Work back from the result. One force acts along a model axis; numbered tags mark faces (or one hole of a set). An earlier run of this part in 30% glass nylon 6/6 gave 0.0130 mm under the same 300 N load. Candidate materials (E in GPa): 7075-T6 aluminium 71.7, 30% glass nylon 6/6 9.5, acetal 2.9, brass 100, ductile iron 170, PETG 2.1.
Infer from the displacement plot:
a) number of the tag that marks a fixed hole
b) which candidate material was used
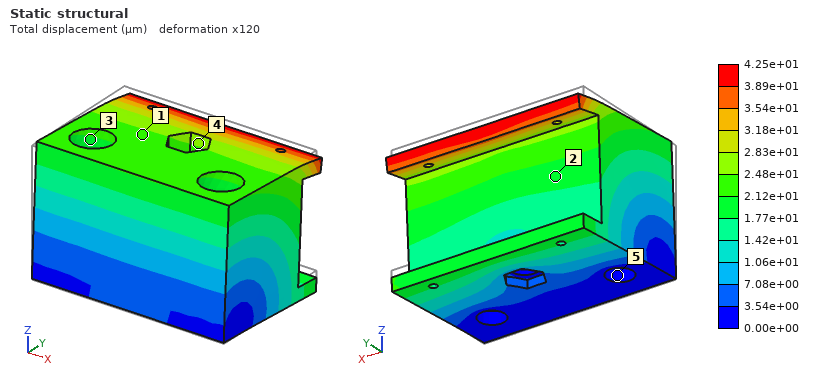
5
acetal
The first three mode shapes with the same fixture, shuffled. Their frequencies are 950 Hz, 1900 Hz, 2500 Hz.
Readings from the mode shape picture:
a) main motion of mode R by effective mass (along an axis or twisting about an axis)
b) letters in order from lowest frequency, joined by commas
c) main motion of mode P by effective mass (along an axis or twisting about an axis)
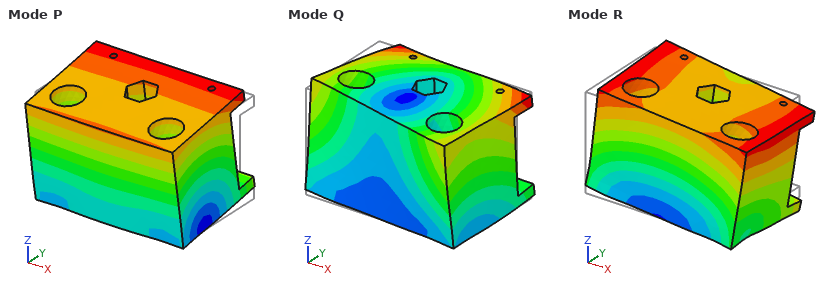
along X
P, R, Q
along Y
